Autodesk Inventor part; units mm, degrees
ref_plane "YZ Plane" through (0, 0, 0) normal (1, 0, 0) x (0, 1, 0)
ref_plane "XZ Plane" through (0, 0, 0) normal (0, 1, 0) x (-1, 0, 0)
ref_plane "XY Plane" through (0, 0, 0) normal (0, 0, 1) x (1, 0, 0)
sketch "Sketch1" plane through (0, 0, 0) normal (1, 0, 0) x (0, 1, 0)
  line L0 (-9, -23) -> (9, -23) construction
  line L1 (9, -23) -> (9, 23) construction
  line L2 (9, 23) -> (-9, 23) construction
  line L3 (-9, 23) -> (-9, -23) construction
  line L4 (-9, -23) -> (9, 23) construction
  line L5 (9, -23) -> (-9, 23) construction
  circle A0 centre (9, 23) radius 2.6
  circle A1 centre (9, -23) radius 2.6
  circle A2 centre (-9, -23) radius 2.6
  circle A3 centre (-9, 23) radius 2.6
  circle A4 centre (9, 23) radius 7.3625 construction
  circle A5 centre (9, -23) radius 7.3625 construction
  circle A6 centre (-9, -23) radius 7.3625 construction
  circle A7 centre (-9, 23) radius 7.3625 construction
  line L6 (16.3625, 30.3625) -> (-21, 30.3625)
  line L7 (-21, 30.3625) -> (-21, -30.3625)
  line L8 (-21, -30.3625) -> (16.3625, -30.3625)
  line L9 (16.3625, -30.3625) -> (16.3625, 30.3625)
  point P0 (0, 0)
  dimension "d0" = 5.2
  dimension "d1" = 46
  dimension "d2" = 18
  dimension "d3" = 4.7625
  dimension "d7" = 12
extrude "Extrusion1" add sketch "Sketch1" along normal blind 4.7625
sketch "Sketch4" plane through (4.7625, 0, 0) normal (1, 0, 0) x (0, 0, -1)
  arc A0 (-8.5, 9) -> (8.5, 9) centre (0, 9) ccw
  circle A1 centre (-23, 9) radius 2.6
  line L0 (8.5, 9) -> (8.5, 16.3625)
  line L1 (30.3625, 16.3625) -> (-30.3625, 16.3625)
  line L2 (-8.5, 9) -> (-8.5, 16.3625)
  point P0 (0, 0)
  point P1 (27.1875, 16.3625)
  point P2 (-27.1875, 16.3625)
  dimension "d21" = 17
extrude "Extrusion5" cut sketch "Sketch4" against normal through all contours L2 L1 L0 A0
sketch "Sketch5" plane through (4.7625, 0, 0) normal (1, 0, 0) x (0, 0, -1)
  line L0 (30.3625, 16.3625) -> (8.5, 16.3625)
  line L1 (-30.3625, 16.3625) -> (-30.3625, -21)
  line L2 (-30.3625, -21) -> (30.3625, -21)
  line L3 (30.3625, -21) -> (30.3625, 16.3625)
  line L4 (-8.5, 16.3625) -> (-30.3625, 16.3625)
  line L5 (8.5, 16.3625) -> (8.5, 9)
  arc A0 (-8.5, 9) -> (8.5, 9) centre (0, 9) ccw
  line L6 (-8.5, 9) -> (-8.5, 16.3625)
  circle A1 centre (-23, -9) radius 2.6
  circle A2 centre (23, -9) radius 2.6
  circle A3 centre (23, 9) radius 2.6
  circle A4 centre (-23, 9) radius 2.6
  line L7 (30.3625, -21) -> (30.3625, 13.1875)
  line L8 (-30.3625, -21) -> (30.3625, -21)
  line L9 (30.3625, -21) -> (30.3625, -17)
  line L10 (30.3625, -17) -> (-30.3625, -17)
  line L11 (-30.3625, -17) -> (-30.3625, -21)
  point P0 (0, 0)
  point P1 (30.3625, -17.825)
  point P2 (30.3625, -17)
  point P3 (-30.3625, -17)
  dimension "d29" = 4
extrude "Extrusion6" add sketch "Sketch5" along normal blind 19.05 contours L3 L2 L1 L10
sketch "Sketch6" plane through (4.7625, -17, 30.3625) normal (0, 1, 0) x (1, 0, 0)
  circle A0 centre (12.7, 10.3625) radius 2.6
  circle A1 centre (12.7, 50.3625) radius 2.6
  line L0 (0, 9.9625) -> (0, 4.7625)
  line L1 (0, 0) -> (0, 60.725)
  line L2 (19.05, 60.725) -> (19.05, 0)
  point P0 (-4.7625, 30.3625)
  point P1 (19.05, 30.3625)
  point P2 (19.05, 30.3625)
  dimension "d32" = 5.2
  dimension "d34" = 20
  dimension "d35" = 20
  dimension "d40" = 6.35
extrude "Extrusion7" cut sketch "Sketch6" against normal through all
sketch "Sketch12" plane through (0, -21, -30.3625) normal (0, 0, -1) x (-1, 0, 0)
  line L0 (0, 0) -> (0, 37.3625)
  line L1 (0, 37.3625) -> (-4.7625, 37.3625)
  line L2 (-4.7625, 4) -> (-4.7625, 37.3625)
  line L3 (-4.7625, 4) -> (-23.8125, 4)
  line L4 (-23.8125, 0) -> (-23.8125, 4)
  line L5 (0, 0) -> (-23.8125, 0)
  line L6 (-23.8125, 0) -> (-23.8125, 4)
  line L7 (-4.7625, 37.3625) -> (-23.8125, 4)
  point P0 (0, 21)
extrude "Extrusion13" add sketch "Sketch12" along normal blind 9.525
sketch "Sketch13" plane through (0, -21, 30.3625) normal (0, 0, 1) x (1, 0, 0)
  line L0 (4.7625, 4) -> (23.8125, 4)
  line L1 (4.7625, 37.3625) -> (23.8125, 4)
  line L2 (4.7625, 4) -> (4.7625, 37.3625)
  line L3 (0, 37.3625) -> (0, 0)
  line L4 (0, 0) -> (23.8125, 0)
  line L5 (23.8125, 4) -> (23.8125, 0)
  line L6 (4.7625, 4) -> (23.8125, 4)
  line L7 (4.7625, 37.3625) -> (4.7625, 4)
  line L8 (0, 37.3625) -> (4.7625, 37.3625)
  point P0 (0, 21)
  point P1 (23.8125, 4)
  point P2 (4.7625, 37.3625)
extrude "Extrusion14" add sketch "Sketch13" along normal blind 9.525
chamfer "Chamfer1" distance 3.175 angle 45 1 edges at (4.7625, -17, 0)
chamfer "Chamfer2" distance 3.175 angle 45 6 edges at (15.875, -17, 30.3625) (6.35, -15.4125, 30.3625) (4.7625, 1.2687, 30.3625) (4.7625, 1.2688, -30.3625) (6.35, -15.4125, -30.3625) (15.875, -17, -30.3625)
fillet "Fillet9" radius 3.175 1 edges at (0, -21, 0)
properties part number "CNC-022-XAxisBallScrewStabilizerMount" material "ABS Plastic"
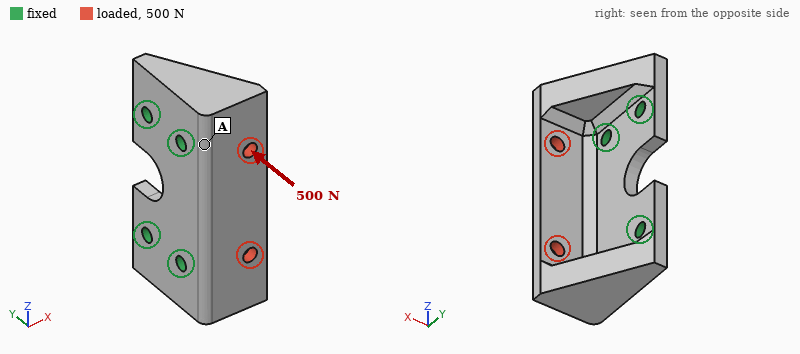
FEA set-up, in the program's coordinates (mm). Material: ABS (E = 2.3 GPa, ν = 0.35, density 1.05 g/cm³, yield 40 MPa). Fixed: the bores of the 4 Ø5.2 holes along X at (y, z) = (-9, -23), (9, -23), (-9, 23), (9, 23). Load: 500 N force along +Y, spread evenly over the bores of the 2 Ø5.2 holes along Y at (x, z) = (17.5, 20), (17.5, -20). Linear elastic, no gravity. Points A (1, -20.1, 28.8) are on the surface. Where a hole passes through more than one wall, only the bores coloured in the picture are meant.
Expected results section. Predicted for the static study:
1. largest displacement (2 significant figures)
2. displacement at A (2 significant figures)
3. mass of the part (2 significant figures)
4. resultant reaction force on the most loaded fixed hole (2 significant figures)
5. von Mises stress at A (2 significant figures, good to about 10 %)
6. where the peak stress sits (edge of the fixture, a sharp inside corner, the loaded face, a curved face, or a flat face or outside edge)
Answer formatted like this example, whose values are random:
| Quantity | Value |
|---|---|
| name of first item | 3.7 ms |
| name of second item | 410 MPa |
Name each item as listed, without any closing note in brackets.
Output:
| Quantity | Value |
|---|---|
| largest displacement | 0.60 mm |
| displacement at A | 0.10 mm |
| mass of the part | 26 g |
| resultant reaction force on the most loaded fixed hole | 230 N |
| von Mises stress at A | 3.8 MPa |
| where the peak stress sits | the loaded face |
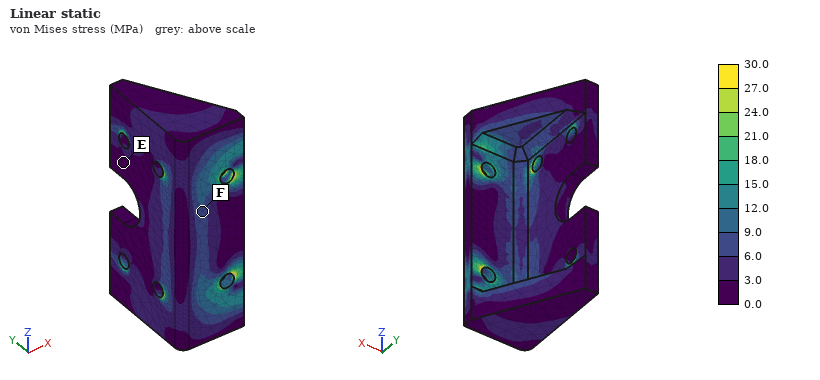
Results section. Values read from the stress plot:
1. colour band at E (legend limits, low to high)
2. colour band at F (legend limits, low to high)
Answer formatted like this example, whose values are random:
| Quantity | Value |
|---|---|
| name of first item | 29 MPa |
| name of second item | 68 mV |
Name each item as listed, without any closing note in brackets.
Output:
| Quantity | Value |
|---|---|
| colour band at E | 0.0 to 3.0 MPa |
| colour band at F | 6.0 to 9.0 MPa |
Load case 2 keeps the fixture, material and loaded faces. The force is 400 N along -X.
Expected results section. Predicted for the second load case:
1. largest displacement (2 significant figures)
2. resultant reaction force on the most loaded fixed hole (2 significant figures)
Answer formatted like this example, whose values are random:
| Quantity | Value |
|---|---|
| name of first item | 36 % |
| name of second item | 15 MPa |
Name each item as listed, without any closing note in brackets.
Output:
| Quantity | Value |
|---|---|
| largest displacement | 0.18 mm |
| resultant reaction force on the most loaded fixed hole | 260 N |
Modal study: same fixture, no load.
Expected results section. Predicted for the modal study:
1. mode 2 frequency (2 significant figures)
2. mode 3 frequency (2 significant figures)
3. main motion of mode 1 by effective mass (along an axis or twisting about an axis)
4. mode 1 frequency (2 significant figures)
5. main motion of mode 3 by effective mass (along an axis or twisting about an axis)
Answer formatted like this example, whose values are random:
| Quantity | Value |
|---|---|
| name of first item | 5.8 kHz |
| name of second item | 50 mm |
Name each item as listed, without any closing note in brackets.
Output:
| Quantity | Value |
|---|---|
| mode 2 frequency | 2700 Hz |
| mode 3 frequency | 3500 Hz |
| main motion of mode 1 by effective mass | along Y |
| mode 1 frequency | 2400 Hz |
| main motion of mode 3 by effective mass | along X |
